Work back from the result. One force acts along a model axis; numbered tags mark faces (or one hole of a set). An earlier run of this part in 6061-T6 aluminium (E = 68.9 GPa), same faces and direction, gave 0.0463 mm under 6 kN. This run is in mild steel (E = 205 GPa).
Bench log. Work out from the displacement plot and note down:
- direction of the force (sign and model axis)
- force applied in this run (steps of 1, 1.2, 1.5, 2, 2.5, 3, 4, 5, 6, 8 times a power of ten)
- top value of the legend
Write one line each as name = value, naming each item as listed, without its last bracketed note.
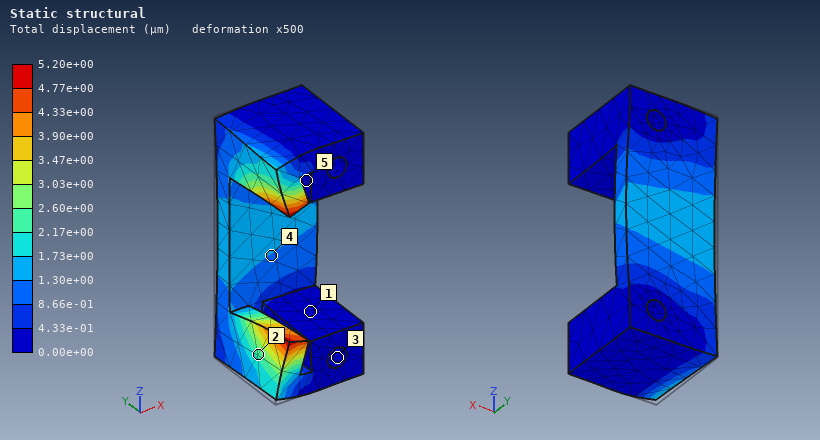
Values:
direction of the force = +X
force applied in this run = 2 kN
top value of the legend = 5.20e+00 µm
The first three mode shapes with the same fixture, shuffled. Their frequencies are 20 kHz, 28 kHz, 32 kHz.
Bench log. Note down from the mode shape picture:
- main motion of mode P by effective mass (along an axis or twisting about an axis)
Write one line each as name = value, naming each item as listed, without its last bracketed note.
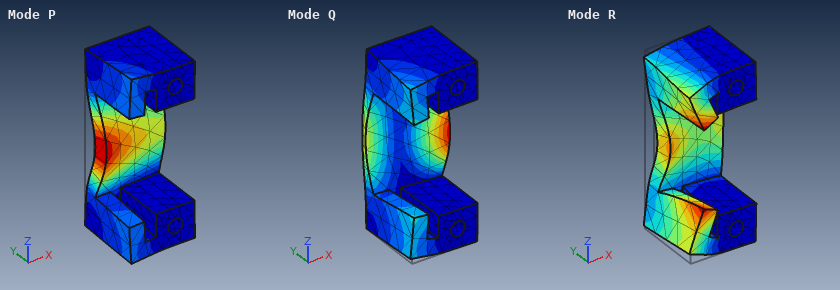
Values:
main motion of mode P by effective mass = along Y
